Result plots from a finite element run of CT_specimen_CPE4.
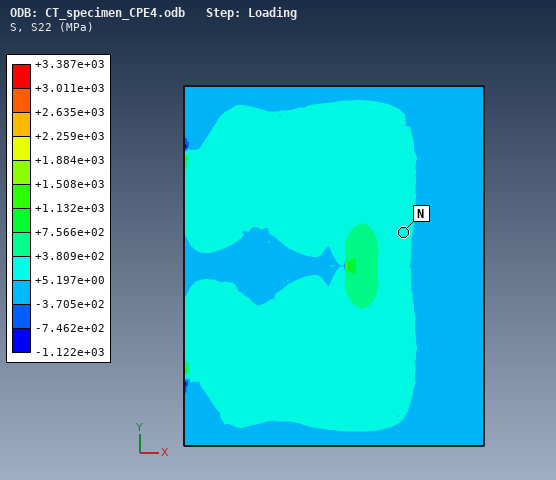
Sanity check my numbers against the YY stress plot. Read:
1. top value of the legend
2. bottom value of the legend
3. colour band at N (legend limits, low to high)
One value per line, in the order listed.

+3.387e+03 MPa
-1.122e+03 MPa
+5.197e+00 to +3.809e+02 MPa
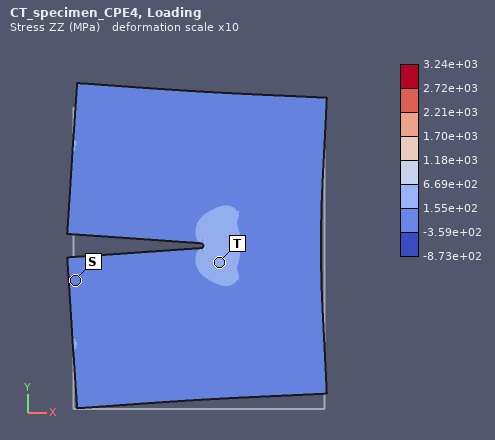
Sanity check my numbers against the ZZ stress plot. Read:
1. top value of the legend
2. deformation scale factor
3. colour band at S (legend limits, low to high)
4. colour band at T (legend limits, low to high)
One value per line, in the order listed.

3.24e+03 MPa
10
-3.59e+02 to 1.55e+02 MPa
1.55e+02 to 6.69e+02 MPa
